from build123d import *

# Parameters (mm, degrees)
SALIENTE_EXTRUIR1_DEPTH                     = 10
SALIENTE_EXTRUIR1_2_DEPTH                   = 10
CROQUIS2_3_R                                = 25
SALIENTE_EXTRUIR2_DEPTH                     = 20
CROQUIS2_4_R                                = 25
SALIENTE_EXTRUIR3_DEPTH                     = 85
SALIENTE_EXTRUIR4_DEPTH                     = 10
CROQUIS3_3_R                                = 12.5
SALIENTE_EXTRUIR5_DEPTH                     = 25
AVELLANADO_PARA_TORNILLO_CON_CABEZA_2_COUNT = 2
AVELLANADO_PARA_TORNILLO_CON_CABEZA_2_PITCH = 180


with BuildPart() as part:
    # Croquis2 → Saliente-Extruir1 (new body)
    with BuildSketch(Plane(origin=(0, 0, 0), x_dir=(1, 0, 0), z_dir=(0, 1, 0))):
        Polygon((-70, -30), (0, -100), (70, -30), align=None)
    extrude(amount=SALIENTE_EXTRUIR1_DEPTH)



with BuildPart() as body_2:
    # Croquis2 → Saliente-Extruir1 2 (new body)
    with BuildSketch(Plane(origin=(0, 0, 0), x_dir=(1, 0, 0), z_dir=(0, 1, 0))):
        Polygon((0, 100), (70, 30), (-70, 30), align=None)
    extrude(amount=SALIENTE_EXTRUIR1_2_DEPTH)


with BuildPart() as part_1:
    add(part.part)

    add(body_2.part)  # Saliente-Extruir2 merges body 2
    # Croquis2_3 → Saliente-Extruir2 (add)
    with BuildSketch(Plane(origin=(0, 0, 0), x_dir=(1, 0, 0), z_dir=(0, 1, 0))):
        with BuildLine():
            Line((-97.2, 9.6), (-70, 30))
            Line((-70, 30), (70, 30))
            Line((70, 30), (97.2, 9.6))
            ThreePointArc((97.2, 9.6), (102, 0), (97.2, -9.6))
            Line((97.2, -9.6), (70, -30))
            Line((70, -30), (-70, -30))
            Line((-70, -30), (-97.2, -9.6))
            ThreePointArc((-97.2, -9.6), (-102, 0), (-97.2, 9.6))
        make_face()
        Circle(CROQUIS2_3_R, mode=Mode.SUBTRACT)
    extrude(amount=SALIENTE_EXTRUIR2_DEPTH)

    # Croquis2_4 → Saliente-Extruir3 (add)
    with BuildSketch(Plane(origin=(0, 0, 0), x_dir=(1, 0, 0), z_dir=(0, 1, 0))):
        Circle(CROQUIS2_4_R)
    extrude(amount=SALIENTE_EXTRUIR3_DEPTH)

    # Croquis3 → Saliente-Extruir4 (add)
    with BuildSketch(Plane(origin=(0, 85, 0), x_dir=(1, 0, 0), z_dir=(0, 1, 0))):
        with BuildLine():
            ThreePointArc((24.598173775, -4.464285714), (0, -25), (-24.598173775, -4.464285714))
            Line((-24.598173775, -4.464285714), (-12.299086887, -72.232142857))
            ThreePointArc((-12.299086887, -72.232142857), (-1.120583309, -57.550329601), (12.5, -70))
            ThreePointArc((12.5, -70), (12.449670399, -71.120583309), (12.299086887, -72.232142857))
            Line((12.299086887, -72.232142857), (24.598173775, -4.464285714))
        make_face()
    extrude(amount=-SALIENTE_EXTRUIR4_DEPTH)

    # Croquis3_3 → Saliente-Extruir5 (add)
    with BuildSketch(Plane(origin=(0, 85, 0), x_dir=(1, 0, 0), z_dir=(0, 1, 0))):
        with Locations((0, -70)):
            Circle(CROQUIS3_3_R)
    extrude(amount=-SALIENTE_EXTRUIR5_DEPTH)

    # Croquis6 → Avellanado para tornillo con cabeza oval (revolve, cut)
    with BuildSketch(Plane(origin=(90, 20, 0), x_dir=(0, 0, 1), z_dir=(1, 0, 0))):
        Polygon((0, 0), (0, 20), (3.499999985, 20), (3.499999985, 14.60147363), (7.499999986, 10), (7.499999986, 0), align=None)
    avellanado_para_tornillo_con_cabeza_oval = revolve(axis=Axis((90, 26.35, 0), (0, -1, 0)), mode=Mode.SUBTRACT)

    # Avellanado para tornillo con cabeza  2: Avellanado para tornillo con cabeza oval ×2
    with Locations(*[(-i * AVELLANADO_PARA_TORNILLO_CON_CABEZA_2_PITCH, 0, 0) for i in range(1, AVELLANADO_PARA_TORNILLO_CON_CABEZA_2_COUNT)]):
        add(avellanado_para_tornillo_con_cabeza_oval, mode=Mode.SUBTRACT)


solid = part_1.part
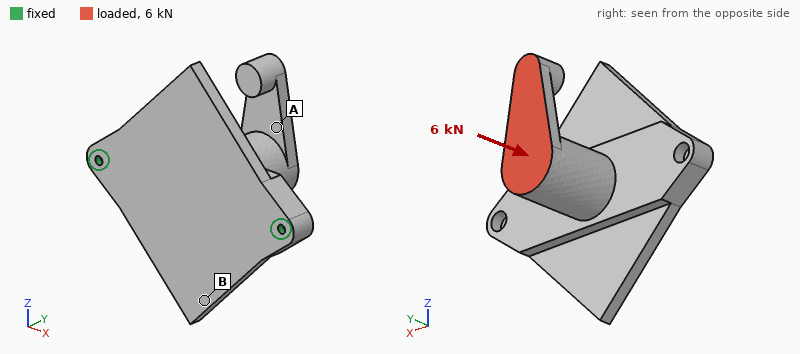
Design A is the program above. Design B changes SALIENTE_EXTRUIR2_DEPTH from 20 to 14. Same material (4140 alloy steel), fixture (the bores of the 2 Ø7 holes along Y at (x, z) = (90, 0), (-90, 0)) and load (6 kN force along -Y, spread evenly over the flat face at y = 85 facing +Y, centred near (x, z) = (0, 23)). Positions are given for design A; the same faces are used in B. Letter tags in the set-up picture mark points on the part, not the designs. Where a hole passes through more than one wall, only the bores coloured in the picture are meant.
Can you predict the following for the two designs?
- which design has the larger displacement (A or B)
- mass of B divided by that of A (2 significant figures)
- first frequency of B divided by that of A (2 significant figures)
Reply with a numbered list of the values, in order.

1. B
2. 0.89
3. 0.88
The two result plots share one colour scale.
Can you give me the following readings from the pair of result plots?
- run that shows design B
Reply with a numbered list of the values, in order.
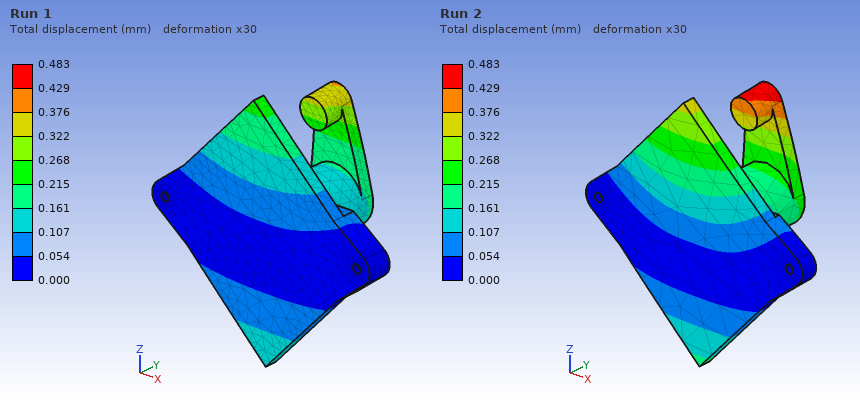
1. Run 2
